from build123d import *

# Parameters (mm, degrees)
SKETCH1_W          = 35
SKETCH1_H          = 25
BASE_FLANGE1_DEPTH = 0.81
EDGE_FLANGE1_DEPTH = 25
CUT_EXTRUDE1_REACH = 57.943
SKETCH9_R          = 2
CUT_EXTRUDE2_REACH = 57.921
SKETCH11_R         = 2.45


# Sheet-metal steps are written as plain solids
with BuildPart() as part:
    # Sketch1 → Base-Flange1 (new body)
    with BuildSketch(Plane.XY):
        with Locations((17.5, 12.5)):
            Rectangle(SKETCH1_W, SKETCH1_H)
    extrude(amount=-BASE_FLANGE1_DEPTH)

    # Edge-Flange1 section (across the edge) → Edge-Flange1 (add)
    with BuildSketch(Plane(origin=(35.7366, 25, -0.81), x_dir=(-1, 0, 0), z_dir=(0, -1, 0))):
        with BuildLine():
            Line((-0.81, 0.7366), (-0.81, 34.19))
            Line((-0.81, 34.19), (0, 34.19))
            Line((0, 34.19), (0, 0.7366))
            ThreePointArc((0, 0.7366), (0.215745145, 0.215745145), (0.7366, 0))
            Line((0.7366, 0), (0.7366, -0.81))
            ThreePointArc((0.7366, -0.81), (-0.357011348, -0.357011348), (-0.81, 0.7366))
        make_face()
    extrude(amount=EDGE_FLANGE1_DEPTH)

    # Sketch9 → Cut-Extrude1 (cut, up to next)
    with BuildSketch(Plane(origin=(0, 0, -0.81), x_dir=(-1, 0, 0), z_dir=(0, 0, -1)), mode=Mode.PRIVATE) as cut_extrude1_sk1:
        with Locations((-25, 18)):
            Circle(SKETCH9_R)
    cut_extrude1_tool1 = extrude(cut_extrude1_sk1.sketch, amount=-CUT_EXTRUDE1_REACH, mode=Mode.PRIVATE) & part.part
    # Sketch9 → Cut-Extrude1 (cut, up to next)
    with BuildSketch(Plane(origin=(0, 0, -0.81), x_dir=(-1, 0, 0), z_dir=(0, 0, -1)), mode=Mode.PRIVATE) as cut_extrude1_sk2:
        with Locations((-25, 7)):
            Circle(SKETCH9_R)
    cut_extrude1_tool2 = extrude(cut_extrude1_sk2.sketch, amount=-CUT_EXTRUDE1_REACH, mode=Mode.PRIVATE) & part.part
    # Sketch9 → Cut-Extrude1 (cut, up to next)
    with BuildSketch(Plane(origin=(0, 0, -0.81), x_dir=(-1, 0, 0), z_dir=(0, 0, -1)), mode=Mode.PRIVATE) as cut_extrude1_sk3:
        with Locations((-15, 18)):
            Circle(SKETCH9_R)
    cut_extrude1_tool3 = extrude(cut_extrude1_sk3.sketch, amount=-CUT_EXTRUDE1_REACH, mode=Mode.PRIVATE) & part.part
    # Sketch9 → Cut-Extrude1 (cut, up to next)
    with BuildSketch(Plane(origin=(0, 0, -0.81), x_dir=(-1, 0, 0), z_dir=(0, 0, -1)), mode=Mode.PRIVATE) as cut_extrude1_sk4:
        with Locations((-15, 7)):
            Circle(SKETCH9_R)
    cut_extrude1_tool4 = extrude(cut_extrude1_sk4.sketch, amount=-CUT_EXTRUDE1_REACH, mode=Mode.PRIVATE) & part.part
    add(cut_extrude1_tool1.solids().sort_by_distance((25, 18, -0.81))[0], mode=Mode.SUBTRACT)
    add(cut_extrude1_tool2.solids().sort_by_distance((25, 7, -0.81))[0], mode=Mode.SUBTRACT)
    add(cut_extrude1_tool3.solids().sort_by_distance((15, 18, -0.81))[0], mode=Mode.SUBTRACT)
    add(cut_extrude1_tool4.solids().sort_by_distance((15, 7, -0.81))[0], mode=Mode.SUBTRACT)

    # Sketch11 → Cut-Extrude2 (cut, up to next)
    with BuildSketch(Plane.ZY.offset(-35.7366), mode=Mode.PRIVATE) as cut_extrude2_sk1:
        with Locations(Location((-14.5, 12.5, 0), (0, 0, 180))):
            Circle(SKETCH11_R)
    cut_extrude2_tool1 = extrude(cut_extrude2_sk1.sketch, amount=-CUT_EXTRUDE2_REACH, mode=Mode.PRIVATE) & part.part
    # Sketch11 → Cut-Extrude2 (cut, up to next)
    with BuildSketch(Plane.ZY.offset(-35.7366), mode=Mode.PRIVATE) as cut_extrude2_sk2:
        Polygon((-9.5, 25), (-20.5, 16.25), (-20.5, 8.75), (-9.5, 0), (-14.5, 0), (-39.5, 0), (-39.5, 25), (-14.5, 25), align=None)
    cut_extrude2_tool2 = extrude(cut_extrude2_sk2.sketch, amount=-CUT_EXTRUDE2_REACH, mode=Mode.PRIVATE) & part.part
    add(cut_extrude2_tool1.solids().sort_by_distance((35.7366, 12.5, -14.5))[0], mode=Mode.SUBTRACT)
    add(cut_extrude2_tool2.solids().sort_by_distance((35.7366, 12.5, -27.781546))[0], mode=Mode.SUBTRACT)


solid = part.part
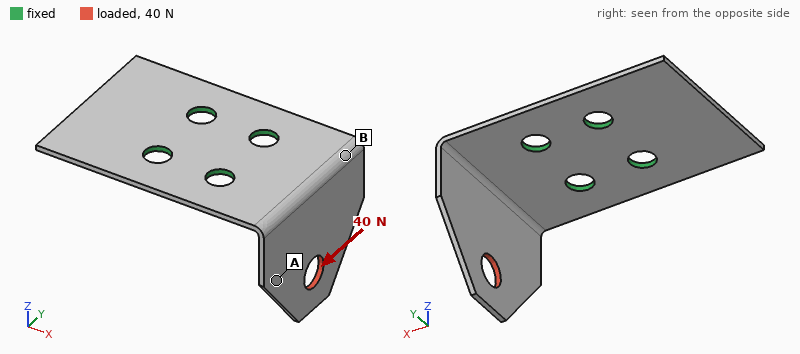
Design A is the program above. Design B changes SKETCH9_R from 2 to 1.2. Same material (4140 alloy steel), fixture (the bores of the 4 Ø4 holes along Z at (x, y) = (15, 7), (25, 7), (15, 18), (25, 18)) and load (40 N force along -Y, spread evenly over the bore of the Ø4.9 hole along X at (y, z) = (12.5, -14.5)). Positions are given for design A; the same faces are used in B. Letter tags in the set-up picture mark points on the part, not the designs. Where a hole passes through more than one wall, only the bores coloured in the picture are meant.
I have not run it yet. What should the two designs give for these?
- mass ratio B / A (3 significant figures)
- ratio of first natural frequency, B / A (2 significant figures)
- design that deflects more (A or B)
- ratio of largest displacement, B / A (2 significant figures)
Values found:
1.03
0.95
B
1.2
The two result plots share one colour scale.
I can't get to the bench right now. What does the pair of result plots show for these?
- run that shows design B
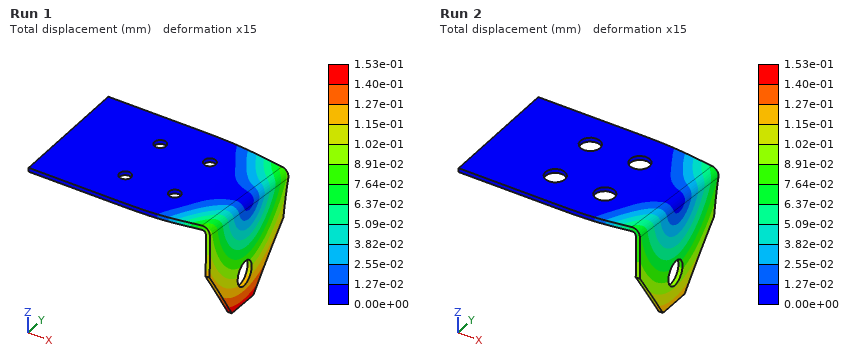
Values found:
Run 1
